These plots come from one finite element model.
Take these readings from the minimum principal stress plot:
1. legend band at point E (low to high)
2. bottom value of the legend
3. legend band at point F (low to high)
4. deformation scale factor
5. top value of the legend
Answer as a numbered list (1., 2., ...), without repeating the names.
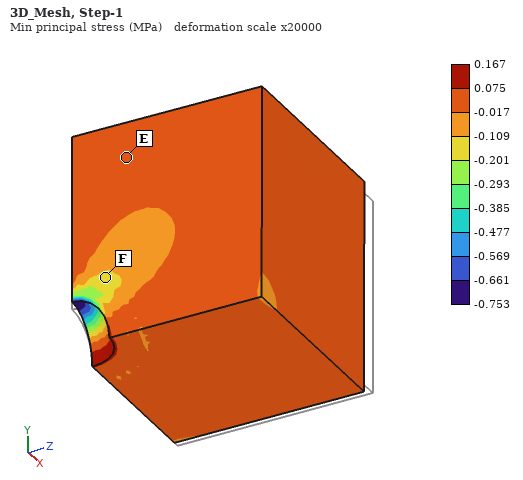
1. -0.017 to 0.075 MPa
2. -0.753 MPa
3. -0.201 to -0.109 MPa
4. 20000
5. 0.167 MPa
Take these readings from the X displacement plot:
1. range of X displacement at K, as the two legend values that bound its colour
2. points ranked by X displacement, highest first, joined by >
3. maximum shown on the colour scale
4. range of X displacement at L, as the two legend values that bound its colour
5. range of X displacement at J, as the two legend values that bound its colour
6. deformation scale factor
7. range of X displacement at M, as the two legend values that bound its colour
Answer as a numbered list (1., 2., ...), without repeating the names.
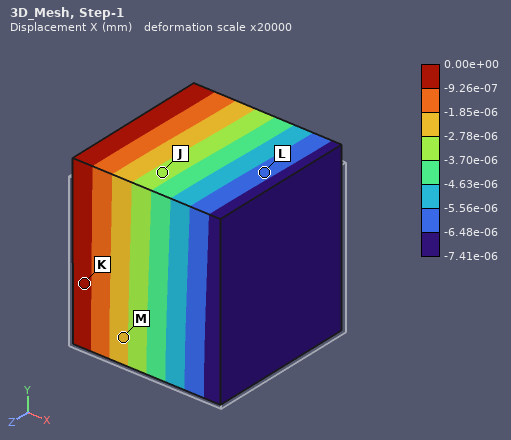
1. -9.26e-07 to 0.00e+00 mm
2. K > M > J > L
3. 0.00e+00 mm
4. -6.48e-06 to -5.56e-06 mm
5. -3.70e-06 to -2.78e-06 mm
6. 20000
7. -2.78e-06 to -1.85e-06 mm
